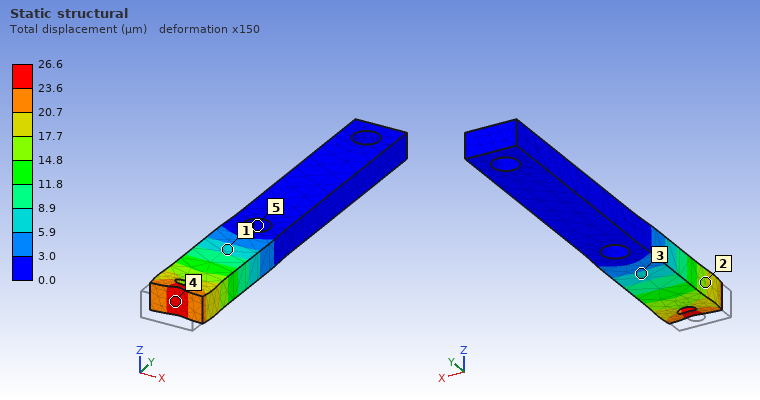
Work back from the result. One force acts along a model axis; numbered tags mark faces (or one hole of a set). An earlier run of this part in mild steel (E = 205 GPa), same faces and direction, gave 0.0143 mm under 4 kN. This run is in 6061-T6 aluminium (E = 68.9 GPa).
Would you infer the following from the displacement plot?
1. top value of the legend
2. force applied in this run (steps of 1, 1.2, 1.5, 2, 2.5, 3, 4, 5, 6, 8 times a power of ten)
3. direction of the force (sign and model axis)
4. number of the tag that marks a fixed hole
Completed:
26.6 µm
2.5 kN
+Y
5
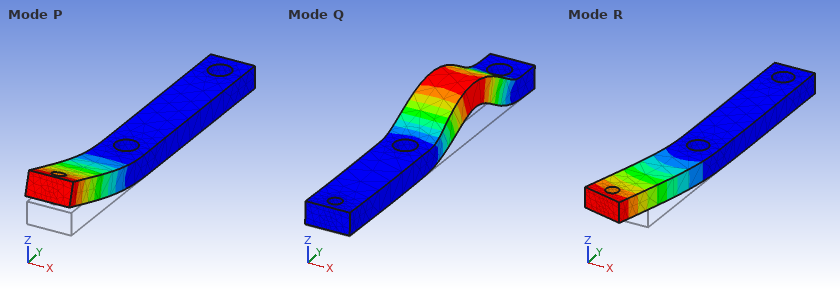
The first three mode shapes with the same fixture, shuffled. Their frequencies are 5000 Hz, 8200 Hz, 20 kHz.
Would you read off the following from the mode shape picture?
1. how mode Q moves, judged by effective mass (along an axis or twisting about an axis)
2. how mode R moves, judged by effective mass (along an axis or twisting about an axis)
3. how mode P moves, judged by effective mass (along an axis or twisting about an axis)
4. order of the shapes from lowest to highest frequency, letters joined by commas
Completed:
along Z
along X
along Z
P, R, Q
